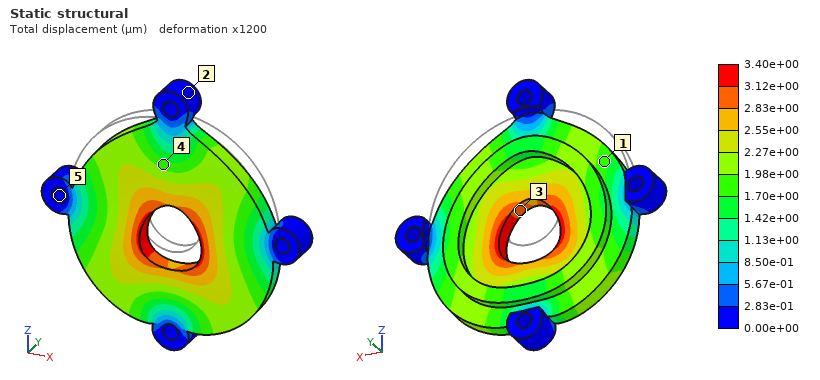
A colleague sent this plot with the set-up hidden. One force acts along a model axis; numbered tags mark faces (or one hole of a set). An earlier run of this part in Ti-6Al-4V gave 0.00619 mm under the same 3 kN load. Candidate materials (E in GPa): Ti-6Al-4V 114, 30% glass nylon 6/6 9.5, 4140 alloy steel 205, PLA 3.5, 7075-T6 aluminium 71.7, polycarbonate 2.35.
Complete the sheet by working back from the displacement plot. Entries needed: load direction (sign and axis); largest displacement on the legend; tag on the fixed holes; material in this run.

-Z
3.40e+00 µm
5
4140 alloy steel
